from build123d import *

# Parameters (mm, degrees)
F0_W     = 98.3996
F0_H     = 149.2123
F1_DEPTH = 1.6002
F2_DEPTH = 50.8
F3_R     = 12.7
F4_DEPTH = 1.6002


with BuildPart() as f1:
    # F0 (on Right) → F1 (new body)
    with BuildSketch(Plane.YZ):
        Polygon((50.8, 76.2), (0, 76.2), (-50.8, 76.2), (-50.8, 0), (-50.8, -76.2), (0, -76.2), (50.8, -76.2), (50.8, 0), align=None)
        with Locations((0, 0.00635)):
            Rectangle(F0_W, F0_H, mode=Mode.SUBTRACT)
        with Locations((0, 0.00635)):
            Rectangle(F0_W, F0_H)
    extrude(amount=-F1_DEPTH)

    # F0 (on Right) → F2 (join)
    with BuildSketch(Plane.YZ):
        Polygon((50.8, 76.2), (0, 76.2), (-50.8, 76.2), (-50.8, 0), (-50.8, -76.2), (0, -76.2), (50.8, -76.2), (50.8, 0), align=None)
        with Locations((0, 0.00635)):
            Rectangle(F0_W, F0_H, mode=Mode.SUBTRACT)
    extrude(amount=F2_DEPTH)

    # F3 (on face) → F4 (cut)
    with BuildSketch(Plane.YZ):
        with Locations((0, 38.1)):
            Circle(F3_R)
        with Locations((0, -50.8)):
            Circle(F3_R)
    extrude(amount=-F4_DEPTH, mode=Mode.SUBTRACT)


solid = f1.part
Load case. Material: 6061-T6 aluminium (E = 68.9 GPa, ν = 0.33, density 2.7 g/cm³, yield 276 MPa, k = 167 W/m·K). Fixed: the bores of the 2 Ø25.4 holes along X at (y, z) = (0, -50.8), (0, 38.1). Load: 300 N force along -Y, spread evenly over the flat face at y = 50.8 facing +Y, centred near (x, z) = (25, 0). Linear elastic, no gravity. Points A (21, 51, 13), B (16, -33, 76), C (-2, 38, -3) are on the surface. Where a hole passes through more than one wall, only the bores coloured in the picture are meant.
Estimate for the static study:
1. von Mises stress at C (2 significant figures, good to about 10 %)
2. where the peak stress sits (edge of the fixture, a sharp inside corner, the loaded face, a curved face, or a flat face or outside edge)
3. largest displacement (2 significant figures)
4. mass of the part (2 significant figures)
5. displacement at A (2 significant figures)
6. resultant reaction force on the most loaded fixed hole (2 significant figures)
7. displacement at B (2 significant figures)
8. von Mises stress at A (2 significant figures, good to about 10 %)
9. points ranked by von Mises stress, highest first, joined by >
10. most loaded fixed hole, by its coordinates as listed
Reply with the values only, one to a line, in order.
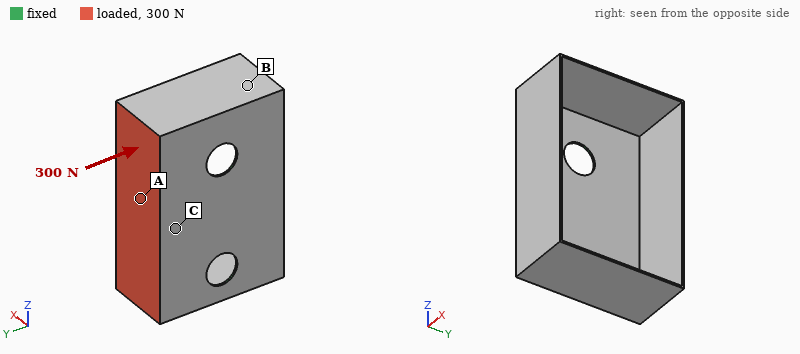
38 MPa
a flat face or outside edge
1.8 mm
170 g
0.81 mm
180 N
0.32 mm
16 MPa
C > A > B
(0, 38.1)
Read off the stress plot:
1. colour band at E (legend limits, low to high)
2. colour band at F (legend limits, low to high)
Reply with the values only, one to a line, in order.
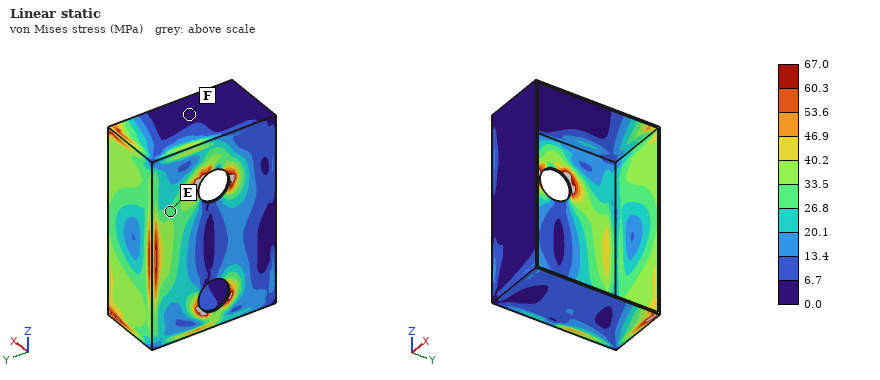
26.8 to 33.5 MPa
0.0 to 6.7 MPa
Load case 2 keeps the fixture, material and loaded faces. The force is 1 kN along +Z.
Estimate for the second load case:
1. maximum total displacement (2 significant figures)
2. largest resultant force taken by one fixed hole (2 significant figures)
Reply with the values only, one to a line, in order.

2.1 mm
710 N
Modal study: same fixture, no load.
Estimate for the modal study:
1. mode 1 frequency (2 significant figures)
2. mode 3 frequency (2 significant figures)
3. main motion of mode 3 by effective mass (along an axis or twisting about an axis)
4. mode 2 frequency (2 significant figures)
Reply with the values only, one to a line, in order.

270 Hz
480 Hz
along X
350 Hz
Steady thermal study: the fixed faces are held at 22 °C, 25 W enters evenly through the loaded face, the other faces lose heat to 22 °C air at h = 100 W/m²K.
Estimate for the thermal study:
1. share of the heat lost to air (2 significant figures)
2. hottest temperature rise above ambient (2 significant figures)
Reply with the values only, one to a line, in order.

78 %
15 K
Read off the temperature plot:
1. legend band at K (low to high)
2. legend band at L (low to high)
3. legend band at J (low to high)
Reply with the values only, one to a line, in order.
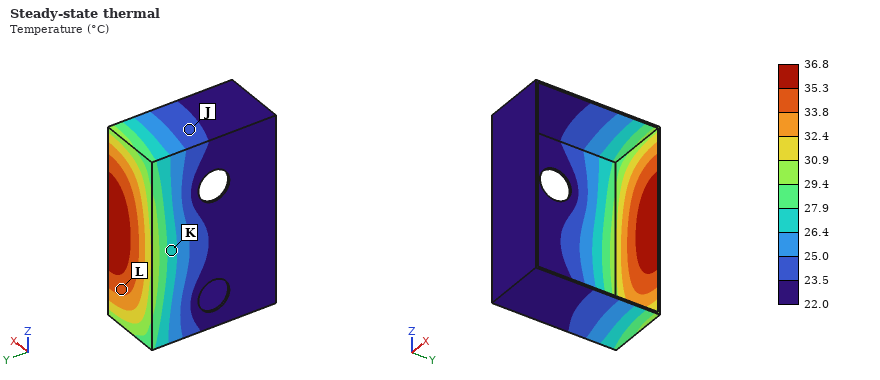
26.4 to 27.9 °C
33.8 to 35.3 °C
23.5 to 25.0 °C
